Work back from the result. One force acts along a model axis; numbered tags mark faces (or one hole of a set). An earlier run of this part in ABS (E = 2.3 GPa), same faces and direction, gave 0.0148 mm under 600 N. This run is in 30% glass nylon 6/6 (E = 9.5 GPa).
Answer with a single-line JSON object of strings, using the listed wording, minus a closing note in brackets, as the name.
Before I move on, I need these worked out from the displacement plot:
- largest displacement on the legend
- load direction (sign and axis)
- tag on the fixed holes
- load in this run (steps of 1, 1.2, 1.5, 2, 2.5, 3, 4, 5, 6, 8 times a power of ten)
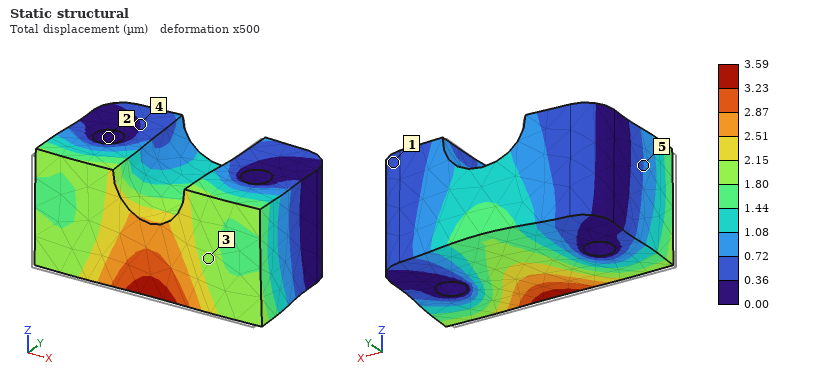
{"largest displacement on the legend": "3.59 µm", "load direction": "+Y", "tag on the fixed holes": "2", "load in this run": "600 N"}
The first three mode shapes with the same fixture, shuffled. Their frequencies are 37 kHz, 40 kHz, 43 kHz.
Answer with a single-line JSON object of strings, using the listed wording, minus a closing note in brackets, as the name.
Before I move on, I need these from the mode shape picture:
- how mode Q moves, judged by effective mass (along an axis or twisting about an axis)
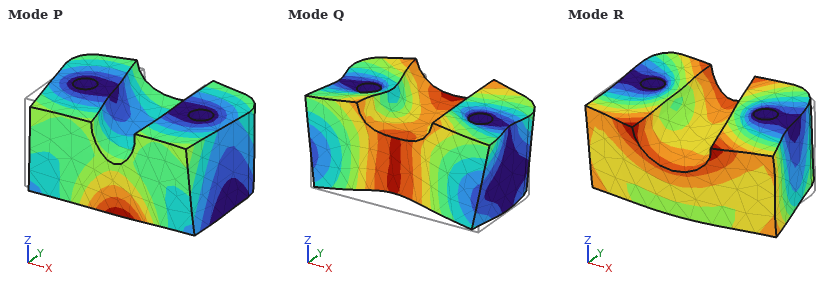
{"how mode Q moves, judged by effective mass": "along Z"}
